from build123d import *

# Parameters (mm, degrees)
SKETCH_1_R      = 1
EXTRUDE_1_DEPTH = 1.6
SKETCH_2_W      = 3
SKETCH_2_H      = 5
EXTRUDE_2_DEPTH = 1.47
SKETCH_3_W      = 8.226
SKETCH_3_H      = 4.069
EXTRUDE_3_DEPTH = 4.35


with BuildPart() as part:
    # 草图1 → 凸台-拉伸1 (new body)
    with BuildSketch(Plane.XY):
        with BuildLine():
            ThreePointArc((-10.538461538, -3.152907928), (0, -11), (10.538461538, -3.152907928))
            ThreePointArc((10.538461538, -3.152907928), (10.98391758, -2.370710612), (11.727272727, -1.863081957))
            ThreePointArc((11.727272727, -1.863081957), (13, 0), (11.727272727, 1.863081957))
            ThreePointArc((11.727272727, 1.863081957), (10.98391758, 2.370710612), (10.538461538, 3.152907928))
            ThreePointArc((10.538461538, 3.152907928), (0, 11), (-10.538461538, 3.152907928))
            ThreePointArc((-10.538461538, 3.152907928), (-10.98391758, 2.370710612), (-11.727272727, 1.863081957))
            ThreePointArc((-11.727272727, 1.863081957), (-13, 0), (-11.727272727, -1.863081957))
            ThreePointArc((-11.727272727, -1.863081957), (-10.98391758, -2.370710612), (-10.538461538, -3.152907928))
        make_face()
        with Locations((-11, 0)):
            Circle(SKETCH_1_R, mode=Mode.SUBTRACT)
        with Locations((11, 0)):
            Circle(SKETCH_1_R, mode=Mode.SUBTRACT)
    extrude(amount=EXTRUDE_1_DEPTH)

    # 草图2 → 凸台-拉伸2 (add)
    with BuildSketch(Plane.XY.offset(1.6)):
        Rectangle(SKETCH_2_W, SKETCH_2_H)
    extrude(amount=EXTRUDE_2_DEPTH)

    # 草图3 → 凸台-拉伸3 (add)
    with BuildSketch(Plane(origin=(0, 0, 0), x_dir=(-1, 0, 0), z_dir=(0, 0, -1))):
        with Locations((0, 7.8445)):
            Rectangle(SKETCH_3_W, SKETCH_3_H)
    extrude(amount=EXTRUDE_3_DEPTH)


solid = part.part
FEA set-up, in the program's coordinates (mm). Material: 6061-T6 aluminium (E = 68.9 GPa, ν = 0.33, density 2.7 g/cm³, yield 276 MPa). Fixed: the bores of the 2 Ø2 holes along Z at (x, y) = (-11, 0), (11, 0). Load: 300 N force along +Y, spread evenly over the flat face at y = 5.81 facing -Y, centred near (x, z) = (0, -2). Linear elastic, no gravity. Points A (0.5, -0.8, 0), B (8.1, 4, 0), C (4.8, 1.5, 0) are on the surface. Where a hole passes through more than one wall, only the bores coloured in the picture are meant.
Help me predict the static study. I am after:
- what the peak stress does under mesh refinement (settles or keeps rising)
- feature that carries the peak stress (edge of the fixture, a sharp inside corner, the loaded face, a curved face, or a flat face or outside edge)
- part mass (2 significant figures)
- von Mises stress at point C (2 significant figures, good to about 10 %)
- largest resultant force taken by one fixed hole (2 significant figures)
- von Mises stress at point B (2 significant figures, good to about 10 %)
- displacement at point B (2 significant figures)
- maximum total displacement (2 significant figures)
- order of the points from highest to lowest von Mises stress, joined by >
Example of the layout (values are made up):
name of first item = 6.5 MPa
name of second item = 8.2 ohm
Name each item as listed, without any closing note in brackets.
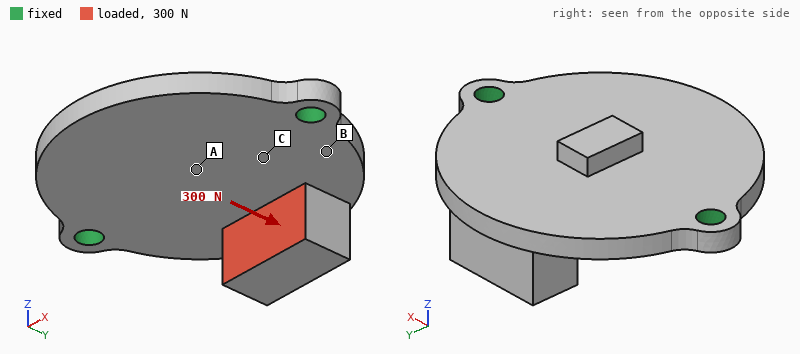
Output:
what the peak stress does under mesh refinement = keeps rising
feature that carries the peak stress = edge of the fixture
part mass = 2.1 g
von Mises stress at point C = 72 MPa
largest resultant force taken by one fixed hole = 150 N
von Mises stress at point B = 110 MPa
displacement at point B = 0.026 mm
maximum total displacement = 0.16 mm
order of the points from highest to lowest von Mises stress, joined by > = B > C > A
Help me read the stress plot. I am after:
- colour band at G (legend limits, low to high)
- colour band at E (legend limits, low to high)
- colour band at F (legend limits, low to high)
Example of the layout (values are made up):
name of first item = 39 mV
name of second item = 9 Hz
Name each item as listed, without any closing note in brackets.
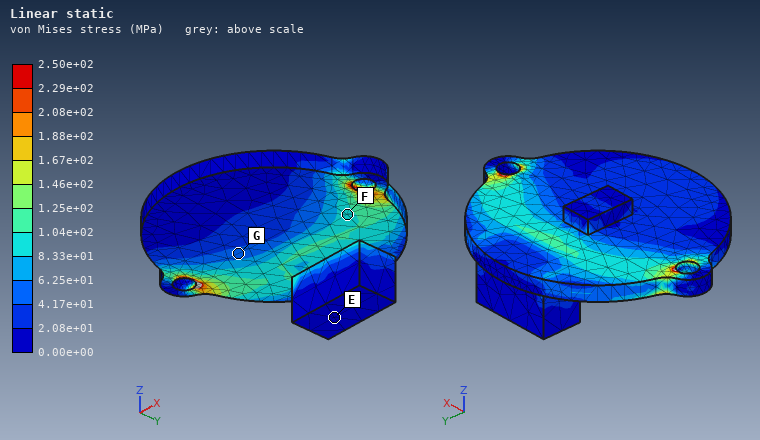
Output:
colour band at G = 4.17e+01 to 6.25e+01 MPa
colour band at E = 0.00e+00 to 2.08e+01 MPa
colour band at F = 8.33e+01 to 1.04e+02 MPa
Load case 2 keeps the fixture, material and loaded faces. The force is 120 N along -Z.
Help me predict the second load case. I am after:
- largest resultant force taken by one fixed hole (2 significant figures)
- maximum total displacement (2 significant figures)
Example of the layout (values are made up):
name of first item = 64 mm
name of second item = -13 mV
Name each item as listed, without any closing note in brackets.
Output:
largest resultant force taken by one fixed hole = 60 N
maximum total displacement = 88 µm
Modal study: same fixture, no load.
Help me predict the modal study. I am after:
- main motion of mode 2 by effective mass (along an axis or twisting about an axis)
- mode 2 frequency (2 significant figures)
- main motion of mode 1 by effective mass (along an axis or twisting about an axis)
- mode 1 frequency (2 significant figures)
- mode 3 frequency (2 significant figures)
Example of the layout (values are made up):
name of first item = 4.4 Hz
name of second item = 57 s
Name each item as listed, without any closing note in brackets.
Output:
main motion of mode 2 by effective mass = along Z
mode 2 frequency = 9800 Hz
main motion of mode 1 by effective mass = along Z
mode 1 frequency = 6000 Hz
mode 3 frequency = 21 kHz
